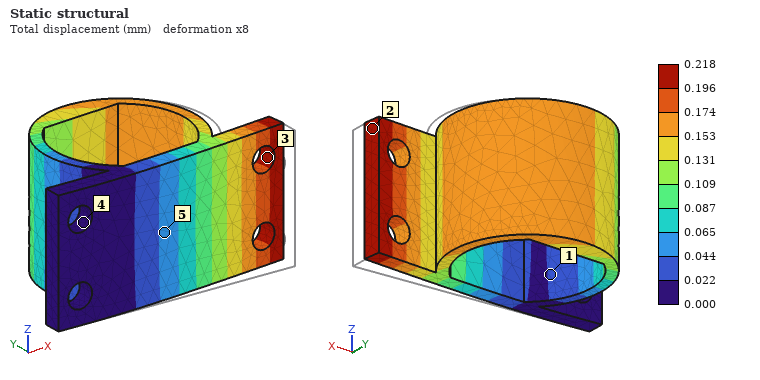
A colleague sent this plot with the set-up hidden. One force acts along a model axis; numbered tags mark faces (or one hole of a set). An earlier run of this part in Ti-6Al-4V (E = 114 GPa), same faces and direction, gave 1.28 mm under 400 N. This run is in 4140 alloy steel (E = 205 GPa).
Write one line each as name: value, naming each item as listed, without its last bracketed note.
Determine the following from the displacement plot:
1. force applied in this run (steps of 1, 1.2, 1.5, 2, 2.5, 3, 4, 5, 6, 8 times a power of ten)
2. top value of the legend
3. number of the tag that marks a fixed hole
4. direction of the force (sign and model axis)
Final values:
force applied in this run: 120 N
top value of the legend: 0.218 mm
number of the tag that marks a fixed hole: 4
direction of the force: +Y
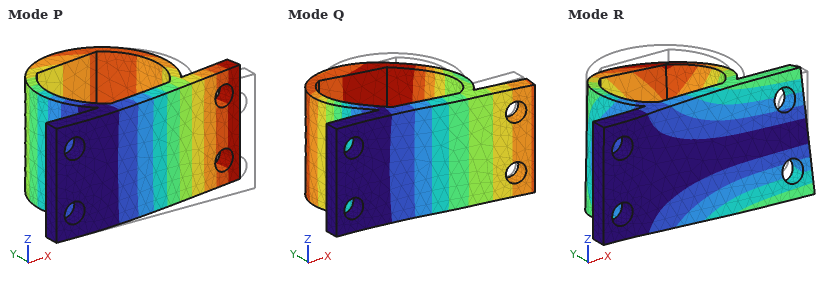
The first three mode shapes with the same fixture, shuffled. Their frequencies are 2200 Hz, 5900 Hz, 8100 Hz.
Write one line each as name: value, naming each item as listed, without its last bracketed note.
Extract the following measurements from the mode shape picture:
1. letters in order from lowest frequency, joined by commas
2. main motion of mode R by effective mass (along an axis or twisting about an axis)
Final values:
letters in order from lowest frequency, joined by commas: P, R, Q
main motion of mode R by effective mass: along Z
